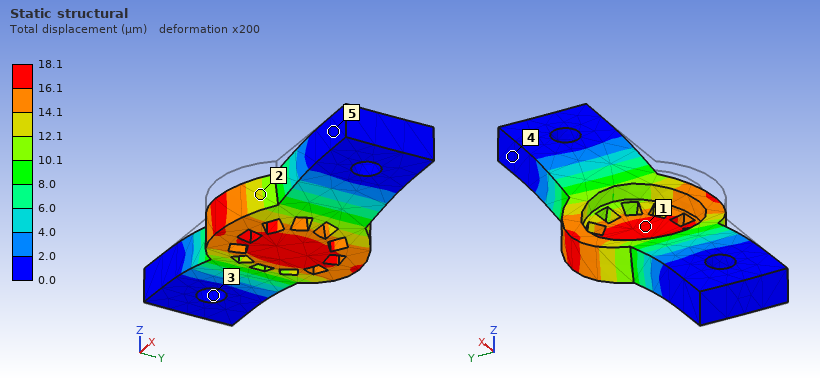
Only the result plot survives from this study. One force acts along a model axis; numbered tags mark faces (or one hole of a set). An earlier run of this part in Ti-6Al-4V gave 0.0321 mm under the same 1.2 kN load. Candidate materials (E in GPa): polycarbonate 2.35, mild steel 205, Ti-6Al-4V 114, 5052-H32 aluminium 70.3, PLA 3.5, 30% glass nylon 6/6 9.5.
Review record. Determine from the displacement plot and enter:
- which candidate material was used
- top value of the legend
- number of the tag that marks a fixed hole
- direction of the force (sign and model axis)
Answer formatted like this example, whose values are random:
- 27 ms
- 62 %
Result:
- mild steel
- 18.1 µm
- 3
- -Z
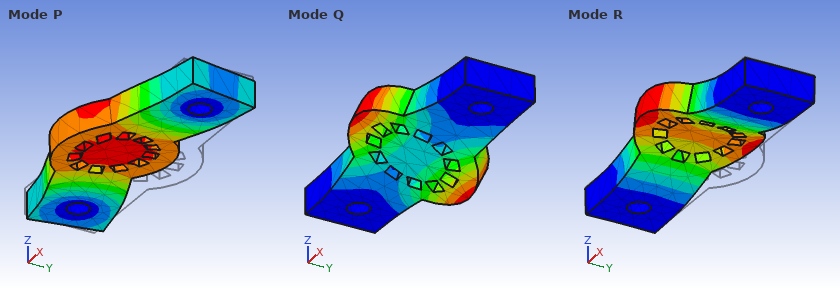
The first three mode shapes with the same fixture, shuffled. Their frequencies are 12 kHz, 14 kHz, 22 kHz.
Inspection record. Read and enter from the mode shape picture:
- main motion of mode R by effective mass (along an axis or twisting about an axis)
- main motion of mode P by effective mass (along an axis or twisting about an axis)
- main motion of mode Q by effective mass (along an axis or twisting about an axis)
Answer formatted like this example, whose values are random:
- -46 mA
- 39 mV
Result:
- along Z
- along Y
- twisting about X
